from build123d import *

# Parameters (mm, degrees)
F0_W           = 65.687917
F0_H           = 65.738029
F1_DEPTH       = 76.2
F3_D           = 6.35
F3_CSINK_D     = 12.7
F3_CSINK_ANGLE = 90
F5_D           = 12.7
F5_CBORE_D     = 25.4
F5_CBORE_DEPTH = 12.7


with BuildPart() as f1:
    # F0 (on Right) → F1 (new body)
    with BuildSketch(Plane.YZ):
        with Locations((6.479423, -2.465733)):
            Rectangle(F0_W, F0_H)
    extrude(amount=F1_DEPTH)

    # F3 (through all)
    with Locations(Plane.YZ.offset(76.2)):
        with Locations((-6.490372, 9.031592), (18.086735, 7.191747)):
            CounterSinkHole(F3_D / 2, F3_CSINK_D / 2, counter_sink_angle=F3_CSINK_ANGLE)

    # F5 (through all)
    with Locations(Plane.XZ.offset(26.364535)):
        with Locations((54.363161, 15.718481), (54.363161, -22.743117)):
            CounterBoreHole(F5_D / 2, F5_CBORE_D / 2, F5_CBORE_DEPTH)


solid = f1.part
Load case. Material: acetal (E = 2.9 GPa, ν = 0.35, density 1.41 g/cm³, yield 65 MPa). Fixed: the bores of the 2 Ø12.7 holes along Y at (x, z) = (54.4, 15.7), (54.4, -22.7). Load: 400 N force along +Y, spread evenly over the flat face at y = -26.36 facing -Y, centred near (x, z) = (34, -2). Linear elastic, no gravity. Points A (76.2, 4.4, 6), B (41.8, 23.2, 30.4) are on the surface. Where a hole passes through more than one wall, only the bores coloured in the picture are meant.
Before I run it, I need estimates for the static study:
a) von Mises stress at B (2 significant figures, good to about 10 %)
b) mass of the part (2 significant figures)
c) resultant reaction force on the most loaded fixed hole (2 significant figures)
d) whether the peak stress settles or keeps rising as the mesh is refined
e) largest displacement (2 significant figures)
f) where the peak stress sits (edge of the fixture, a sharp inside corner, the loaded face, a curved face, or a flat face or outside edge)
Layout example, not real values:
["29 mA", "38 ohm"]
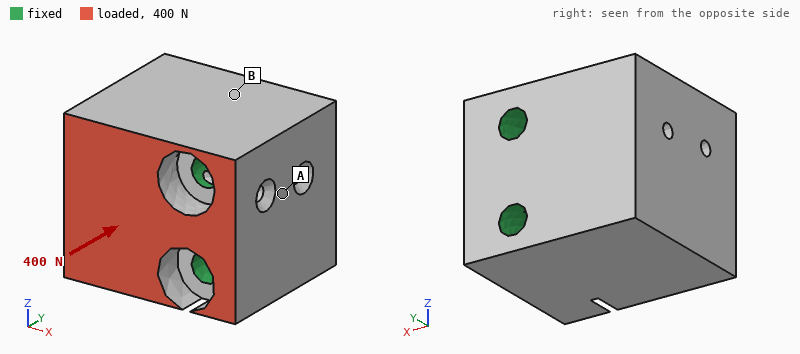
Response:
["0.13 MPa", "420 g", "200 N", "keeps rising", "7.3 µm", "edge of the fixture"]
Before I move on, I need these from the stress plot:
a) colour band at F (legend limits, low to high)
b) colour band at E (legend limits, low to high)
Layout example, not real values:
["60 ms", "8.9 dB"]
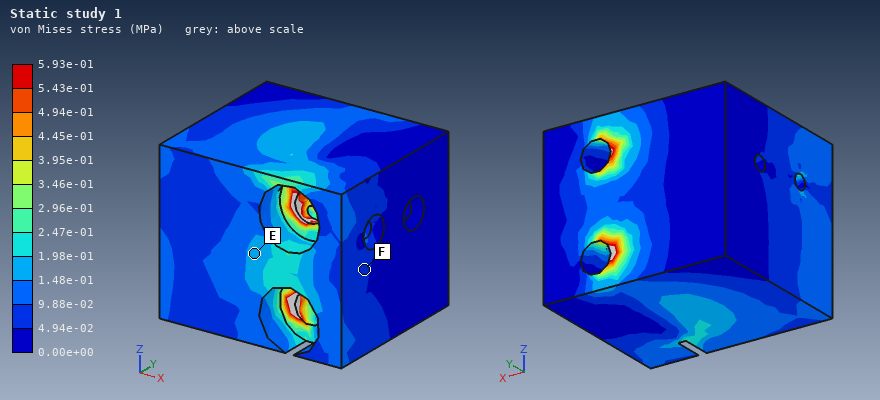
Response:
["4.94e-02 to 9.88e-02 MPa", "1.48e-01 to 1.98e-01 MPa"]
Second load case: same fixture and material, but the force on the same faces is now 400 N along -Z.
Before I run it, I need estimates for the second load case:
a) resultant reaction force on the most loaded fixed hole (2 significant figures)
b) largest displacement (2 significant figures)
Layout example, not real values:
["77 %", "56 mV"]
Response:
["330 N", "13 µm"]
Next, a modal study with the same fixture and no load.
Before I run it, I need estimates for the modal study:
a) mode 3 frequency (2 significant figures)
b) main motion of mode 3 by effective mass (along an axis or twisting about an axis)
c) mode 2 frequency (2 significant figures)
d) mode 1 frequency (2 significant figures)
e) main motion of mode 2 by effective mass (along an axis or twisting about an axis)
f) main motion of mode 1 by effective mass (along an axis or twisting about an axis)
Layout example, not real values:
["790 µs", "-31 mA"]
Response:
["3600 Hz", "twisting about X", "2800 Hz", "2500 Hz", "along Z", "along Y"]
